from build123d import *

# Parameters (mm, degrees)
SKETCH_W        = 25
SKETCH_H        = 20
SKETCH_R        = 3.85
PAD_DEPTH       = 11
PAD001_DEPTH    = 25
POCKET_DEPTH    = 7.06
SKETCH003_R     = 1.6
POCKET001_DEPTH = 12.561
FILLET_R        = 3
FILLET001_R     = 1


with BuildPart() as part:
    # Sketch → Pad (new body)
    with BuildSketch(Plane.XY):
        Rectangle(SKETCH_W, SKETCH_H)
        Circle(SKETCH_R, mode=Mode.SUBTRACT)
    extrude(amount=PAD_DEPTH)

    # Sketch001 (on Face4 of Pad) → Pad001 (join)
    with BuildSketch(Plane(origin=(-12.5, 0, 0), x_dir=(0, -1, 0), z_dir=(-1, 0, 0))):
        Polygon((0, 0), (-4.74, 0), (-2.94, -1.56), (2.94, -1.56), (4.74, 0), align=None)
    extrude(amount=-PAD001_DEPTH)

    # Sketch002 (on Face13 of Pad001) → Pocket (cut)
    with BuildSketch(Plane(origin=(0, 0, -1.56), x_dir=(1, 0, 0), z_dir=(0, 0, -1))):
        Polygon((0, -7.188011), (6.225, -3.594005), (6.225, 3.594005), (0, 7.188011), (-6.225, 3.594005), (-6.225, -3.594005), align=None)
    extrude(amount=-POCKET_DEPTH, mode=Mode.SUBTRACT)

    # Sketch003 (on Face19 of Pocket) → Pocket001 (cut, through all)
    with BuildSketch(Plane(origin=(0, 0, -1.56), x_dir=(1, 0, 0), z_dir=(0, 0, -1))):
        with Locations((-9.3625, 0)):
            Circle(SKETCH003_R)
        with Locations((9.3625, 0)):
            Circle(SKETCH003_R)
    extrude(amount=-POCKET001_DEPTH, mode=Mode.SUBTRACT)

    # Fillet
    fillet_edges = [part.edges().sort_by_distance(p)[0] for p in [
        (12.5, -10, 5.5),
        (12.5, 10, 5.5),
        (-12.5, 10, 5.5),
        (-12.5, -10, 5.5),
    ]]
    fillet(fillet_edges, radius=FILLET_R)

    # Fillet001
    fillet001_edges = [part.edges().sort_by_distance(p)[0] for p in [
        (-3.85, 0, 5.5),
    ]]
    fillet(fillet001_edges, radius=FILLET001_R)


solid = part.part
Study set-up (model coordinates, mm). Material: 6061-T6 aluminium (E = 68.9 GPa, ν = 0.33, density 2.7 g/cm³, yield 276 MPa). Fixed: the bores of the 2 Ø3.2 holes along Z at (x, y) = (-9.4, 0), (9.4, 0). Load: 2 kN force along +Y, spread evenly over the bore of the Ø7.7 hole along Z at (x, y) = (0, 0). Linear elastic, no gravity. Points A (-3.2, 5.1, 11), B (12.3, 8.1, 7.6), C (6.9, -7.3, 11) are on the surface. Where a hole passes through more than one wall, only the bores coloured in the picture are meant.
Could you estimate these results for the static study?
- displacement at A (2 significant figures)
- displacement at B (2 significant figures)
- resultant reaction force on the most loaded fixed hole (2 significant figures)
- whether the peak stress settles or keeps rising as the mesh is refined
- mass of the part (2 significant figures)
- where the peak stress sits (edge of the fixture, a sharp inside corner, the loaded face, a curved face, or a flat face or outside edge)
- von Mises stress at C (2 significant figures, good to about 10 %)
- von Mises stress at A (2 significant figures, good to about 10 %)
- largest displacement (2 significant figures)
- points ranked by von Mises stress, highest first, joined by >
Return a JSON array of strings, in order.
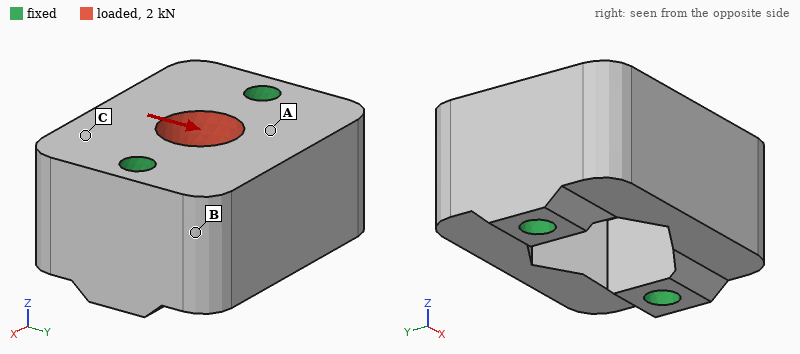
["3.2 µm", "1.0 µm", "1.0 kN", "keeps rising", "12 g", "edge of the fixture", "12 MPa", "21 MPa", "4.5 µm", "A > C > B"]
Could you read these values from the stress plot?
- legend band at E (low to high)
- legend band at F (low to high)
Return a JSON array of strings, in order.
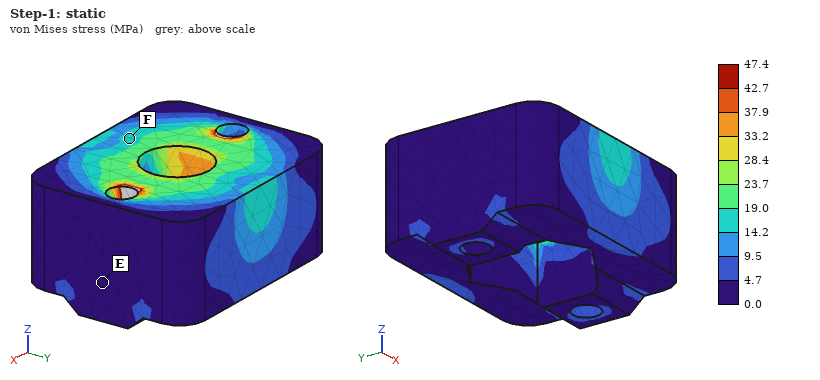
["0.0 to 4.7 MPa", "14.2 to 19.0 MPa"]
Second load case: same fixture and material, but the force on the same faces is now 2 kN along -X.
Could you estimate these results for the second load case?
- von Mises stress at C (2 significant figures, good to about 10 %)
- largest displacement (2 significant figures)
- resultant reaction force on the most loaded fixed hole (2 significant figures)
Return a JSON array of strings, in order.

["3.3 MPa", "2.6 µm", "1.0 kN"]
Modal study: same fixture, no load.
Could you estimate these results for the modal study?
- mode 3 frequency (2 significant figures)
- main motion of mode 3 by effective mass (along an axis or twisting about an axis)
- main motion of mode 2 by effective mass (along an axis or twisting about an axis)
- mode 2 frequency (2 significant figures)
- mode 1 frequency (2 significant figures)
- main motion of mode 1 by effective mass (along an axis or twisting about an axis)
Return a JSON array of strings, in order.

["52 kHz", "twisting about Z", "along Z", "49 kHz", "47 kHz", "twisting about X"]
